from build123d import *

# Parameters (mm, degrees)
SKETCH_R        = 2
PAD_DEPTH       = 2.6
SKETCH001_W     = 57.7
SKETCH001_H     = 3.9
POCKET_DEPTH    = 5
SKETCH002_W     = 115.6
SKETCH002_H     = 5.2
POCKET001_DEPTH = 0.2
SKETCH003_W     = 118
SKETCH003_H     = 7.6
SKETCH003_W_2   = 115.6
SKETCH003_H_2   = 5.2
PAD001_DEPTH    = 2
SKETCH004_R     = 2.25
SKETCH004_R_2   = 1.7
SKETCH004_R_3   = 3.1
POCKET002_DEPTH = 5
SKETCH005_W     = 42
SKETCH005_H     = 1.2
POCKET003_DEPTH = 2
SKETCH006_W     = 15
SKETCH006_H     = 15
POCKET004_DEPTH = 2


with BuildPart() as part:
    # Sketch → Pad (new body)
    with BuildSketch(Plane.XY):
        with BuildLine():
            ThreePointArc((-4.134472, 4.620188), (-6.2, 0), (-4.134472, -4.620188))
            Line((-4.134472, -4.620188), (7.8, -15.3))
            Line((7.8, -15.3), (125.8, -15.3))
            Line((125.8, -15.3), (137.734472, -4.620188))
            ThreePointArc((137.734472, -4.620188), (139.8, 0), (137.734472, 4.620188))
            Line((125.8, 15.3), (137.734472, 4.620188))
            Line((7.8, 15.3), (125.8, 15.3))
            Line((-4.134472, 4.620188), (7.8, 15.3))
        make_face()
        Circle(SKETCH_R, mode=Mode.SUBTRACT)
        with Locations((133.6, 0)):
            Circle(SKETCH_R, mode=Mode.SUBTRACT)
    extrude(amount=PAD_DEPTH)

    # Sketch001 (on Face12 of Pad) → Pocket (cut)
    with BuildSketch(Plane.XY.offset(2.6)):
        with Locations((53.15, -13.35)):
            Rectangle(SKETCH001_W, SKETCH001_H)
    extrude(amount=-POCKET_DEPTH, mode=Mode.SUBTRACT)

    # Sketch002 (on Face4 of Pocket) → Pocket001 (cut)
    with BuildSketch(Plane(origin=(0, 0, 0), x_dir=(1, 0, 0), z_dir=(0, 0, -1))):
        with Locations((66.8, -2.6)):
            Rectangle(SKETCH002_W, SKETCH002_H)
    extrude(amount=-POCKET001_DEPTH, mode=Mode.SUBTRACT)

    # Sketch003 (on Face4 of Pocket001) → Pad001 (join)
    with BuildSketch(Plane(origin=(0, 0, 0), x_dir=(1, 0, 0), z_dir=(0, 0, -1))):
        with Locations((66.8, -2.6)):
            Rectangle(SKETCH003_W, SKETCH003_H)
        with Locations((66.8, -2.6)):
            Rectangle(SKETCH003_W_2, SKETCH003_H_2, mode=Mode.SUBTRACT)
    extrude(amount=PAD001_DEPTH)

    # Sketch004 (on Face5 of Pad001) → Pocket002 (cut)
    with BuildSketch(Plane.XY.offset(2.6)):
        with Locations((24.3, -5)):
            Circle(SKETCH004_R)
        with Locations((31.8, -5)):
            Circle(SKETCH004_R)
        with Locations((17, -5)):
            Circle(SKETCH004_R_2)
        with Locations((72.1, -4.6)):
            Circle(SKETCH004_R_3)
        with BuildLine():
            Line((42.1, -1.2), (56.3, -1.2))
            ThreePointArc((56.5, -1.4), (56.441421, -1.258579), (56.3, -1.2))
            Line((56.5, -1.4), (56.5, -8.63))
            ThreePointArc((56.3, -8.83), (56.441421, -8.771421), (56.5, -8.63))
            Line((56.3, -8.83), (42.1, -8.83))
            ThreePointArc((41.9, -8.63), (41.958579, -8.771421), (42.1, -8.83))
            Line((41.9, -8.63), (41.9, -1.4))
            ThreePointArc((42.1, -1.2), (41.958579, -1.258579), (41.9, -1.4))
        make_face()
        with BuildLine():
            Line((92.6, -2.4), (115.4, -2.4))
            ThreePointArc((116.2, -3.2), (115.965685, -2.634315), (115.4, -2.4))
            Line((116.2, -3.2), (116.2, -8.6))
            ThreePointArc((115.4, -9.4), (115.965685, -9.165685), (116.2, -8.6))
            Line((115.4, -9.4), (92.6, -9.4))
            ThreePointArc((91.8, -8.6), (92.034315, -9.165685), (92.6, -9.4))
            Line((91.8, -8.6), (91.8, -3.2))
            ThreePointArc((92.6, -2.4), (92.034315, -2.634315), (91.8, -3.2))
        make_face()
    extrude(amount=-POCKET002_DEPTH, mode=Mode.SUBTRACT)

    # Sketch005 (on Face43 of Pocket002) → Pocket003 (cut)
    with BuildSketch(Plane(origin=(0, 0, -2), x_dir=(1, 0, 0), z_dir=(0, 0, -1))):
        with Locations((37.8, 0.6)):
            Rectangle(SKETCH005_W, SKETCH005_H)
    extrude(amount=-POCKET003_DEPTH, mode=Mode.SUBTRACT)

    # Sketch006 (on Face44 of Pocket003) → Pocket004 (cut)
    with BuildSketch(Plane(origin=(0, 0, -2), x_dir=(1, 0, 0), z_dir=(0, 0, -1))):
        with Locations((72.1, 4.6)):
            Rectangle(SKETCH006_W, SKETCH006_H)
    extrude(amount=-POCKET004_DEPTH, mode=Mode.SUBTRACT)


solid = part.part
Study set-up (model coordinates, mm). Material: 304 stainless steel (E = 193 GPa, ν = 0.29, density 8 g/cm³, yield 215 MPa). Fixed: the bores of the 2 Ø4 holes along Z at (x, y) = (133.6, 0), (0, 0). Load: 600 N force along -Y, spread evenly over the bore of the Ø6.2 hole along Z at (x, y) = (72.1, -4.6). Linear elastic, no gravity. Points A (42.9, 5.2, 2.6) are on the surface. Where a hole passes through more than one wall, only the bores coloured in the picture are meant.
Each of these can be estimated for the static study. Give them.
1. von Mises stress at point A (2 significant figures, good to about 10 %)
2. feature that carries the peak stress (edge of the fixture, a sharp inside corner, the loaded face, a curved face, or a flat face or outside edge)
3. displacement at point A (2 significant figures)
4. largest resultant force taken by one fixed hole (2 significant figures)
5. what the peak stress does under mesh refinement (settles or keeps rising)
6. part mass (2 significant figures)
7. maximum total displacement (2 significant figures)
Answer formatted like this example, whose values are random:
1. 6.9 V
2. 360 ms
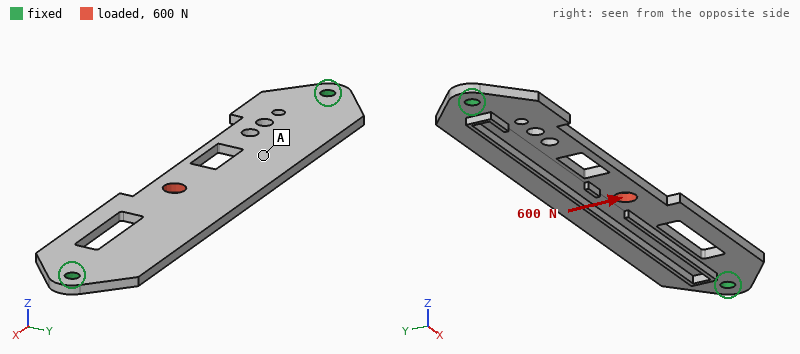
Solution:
1. 15 MPa
2. edge of the fixture
3. 25 µm
4. 430 N
5. keeps rising
6. 76 g
7. 34 µm
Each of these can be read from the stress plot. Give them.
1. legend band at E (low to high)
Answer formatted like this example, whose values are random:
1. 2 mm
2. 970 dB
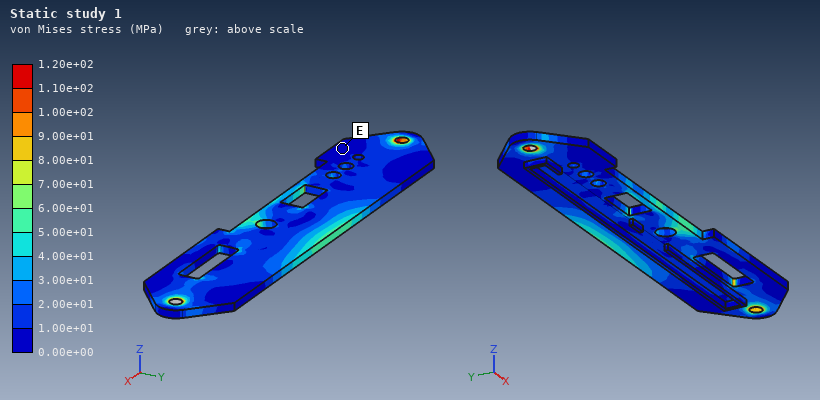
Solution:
1. 0.00e+00 to 1.00e+01 MPa
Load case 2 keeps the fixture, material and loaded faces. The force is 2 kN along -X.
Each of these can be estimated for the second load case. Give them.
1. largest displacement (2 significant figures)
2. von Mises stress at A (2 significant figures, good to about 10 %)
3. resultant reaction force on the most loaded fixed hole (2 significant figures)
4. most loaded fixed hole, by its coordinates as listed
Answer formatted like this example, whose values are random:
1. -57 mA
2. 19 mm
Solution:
1. 11 µm
2. 16 MPa
3. 1.2 kN
4. (133.6, 0)
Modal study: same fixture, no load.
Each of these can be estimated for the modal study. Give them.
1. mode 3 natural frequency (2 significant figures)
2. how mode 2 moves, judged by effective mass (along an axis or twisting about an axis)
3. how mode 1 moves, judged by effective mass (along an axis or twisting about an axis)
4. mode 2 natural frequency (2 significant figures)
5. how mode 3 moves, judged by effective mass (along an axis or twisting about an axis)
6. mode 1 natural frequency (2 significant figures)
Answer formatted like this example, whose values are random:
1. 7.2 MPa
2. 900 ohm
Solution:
1. 2200 Hz
2. twisting about X
3. along Z
4. 1900 Hz
5. twisting about Y
6. 760 Hz
